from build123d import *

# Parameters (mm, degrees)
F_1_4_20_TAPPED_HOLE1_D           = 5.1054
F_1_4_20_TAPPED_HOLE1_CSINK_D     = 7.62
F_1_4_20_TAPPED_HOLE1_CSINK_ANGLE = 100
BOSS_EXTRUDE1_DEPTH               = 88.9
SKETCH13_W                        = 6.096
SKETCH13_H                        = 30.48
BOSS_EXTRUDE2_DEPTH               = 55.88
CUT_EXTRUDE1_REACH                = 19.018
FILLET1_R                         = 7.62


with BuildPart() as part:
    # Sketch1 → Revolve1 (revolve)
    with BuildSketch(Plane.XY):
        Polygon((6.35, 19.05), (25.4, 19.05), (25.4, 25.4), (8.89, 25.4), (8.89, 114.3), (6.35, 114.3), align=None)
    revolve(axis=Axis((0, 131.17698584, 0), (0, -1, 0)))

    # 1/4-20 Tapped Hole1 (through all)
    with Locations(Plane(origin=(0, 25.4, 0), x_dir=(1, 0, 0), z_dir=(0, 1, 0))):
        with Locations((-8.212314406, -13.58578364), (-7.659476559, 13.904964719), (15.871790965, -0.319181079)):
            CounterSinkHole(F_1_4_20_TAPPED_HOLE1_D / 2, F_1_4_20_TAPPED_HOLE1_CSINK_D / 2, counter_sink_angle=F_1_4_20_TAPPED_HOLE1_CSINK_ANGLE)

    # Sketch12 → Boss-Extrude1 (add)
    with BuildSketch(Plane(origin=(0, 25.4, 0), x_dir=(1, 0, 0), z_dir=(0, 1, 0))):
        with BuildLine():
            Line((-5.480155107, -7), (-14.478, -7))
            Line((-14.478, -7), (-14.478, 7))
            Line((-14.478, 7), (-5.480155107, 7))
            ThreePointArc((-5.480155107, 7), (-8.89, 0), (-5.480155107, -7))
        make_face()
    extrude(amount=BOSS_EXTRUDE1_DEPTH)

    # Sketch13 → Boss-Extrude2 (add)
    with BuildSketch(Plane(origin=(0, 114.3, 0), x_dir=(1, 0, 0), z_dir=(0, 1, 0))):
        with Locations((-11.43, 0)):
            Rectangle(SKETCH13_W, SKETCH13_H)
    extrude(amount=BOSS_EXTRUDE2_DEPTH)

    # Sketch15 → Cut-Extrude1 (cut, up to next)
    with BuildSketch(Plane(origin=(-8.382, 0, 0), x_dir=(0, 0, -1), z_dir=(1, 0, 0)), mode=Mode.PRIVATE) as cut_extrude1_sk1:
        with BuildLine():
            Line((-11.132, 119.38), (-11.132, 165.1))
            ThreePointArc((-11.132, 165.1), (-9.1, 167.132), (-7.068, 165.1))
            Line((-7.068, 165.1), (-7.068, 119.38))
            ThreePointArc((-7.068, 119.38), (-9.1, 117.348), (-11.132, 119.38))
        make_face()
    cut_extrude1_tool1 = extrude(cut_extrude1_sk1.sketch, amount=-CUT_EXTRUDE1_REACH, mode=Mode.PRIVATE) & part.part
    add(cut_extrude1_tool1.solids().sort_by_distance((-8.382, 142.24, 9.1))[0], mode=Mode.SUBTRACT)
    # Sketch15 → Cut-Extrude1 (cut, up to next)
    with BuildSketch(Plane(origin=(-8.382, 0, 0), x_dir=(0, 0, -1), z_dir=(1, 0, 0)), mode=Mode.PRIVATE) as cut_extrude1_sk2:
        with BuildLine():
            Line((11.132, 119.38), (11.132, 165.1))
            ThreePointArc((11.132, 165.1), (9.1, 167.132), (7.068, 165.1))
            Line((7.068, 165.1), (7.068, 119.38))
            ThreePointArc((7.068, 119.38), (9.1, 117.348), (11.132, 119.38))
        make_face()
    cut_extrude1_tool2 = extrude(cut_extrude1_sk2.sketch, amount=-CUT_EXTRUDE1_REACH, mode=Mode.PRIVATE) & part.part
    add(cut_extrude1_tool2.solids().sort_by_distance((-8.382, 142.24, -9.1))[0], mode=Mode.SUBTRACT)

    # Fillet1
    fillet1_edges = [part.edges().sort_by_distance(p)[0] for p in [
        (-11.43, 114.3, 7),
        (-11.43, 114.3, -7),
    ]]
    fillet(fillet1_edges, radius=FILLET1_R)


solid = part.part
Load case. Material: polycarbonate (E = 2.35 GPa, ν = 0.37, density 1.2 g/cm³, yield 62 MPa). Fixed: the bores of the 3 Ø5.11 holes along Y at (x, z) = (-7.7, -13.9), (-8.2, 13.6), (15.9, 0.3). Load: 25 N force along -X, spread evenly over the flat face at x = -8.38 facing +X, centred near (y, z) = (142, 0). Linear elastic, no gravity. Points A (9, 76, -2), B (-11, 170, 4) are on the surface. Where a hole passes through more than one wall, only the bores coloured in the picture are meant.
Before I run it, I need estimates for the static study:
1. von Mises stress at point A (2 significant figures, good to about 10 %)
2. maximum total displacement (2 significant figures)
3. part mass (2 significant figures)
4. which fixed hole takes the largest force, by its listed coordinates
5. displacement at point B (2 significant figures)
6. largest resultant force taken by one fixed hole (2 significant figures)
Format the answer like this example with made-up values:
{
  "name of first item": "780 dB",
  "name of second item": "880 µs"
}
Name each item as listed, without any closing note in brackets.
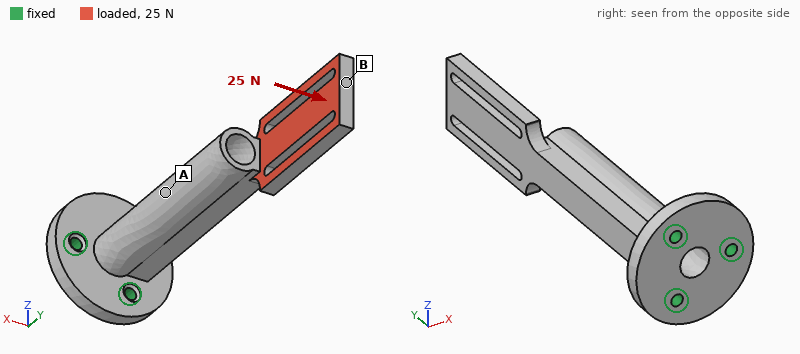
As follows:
{
  "von Mises stress at point A": "2.1 MPa",
  "maximum total displacement": "1.9 mm",
  "part mass": "47 g",
  "which fixed hole takes the largest force, by its listed coordinates": "(15.9, 0.3)",
  "displacement at point B": "1.9 mm",
  "largest resultant force taken by one fixed hole": "110 N"
}
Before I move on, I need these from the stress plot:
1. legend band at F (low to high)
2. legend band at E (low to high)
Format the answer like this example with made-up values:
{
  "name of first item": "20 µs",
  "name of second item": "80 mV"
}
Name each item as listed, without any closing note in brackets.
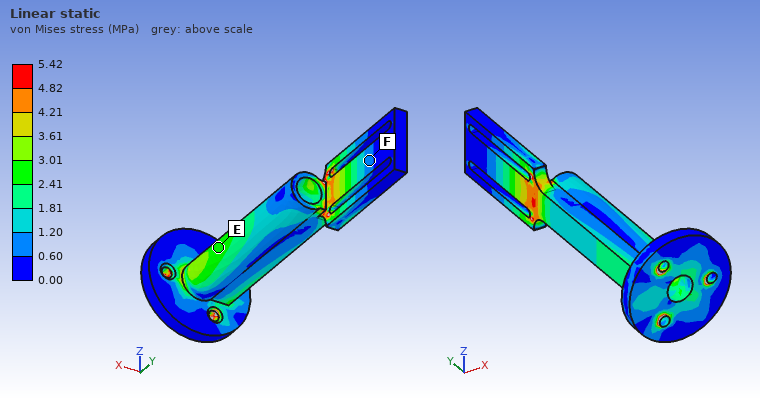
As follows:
{
  "legend band at F": "0.60 to 1.20 MPa",
  "legend band at E": "2.41 to 3.01 MPa"
}
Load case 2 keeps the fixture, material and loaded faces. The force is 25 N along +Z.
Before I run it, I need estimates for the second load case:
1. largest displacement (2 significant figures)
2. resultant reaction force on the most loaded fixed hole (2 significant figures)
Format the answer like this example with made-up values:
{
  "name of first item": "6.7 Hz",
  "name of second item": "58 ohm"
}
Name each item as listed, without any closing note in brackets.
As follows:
{
  "largest displacement": "1.9 mm",
  "resultant reaction force on the most loaded fixed hole": "120 N"
}
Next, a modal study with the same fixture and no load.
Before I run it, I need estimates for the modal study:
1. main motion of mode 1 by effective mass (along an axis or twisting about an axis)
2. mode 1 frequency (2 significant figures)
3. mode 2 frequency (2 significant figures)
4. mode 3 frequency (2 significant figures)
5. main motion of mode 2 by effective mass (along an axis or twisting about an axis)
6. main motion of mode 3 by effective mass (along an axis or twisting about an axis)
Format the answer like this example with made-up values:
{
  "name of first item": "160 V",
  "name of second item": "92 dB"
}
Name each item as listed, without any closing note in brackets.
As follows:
{
  "main motion of mode 1 by effective mass": "along Z",
  "mode 1 frequency": "190 Hz",
  "mode 2 frequency": "210 Hz",
  "mode 3 frequency": "590 Hz",
  "main motion of mode 2 by effective mass": "along X",
  "main motion of mode 3 by effective mass": "along X"
}
